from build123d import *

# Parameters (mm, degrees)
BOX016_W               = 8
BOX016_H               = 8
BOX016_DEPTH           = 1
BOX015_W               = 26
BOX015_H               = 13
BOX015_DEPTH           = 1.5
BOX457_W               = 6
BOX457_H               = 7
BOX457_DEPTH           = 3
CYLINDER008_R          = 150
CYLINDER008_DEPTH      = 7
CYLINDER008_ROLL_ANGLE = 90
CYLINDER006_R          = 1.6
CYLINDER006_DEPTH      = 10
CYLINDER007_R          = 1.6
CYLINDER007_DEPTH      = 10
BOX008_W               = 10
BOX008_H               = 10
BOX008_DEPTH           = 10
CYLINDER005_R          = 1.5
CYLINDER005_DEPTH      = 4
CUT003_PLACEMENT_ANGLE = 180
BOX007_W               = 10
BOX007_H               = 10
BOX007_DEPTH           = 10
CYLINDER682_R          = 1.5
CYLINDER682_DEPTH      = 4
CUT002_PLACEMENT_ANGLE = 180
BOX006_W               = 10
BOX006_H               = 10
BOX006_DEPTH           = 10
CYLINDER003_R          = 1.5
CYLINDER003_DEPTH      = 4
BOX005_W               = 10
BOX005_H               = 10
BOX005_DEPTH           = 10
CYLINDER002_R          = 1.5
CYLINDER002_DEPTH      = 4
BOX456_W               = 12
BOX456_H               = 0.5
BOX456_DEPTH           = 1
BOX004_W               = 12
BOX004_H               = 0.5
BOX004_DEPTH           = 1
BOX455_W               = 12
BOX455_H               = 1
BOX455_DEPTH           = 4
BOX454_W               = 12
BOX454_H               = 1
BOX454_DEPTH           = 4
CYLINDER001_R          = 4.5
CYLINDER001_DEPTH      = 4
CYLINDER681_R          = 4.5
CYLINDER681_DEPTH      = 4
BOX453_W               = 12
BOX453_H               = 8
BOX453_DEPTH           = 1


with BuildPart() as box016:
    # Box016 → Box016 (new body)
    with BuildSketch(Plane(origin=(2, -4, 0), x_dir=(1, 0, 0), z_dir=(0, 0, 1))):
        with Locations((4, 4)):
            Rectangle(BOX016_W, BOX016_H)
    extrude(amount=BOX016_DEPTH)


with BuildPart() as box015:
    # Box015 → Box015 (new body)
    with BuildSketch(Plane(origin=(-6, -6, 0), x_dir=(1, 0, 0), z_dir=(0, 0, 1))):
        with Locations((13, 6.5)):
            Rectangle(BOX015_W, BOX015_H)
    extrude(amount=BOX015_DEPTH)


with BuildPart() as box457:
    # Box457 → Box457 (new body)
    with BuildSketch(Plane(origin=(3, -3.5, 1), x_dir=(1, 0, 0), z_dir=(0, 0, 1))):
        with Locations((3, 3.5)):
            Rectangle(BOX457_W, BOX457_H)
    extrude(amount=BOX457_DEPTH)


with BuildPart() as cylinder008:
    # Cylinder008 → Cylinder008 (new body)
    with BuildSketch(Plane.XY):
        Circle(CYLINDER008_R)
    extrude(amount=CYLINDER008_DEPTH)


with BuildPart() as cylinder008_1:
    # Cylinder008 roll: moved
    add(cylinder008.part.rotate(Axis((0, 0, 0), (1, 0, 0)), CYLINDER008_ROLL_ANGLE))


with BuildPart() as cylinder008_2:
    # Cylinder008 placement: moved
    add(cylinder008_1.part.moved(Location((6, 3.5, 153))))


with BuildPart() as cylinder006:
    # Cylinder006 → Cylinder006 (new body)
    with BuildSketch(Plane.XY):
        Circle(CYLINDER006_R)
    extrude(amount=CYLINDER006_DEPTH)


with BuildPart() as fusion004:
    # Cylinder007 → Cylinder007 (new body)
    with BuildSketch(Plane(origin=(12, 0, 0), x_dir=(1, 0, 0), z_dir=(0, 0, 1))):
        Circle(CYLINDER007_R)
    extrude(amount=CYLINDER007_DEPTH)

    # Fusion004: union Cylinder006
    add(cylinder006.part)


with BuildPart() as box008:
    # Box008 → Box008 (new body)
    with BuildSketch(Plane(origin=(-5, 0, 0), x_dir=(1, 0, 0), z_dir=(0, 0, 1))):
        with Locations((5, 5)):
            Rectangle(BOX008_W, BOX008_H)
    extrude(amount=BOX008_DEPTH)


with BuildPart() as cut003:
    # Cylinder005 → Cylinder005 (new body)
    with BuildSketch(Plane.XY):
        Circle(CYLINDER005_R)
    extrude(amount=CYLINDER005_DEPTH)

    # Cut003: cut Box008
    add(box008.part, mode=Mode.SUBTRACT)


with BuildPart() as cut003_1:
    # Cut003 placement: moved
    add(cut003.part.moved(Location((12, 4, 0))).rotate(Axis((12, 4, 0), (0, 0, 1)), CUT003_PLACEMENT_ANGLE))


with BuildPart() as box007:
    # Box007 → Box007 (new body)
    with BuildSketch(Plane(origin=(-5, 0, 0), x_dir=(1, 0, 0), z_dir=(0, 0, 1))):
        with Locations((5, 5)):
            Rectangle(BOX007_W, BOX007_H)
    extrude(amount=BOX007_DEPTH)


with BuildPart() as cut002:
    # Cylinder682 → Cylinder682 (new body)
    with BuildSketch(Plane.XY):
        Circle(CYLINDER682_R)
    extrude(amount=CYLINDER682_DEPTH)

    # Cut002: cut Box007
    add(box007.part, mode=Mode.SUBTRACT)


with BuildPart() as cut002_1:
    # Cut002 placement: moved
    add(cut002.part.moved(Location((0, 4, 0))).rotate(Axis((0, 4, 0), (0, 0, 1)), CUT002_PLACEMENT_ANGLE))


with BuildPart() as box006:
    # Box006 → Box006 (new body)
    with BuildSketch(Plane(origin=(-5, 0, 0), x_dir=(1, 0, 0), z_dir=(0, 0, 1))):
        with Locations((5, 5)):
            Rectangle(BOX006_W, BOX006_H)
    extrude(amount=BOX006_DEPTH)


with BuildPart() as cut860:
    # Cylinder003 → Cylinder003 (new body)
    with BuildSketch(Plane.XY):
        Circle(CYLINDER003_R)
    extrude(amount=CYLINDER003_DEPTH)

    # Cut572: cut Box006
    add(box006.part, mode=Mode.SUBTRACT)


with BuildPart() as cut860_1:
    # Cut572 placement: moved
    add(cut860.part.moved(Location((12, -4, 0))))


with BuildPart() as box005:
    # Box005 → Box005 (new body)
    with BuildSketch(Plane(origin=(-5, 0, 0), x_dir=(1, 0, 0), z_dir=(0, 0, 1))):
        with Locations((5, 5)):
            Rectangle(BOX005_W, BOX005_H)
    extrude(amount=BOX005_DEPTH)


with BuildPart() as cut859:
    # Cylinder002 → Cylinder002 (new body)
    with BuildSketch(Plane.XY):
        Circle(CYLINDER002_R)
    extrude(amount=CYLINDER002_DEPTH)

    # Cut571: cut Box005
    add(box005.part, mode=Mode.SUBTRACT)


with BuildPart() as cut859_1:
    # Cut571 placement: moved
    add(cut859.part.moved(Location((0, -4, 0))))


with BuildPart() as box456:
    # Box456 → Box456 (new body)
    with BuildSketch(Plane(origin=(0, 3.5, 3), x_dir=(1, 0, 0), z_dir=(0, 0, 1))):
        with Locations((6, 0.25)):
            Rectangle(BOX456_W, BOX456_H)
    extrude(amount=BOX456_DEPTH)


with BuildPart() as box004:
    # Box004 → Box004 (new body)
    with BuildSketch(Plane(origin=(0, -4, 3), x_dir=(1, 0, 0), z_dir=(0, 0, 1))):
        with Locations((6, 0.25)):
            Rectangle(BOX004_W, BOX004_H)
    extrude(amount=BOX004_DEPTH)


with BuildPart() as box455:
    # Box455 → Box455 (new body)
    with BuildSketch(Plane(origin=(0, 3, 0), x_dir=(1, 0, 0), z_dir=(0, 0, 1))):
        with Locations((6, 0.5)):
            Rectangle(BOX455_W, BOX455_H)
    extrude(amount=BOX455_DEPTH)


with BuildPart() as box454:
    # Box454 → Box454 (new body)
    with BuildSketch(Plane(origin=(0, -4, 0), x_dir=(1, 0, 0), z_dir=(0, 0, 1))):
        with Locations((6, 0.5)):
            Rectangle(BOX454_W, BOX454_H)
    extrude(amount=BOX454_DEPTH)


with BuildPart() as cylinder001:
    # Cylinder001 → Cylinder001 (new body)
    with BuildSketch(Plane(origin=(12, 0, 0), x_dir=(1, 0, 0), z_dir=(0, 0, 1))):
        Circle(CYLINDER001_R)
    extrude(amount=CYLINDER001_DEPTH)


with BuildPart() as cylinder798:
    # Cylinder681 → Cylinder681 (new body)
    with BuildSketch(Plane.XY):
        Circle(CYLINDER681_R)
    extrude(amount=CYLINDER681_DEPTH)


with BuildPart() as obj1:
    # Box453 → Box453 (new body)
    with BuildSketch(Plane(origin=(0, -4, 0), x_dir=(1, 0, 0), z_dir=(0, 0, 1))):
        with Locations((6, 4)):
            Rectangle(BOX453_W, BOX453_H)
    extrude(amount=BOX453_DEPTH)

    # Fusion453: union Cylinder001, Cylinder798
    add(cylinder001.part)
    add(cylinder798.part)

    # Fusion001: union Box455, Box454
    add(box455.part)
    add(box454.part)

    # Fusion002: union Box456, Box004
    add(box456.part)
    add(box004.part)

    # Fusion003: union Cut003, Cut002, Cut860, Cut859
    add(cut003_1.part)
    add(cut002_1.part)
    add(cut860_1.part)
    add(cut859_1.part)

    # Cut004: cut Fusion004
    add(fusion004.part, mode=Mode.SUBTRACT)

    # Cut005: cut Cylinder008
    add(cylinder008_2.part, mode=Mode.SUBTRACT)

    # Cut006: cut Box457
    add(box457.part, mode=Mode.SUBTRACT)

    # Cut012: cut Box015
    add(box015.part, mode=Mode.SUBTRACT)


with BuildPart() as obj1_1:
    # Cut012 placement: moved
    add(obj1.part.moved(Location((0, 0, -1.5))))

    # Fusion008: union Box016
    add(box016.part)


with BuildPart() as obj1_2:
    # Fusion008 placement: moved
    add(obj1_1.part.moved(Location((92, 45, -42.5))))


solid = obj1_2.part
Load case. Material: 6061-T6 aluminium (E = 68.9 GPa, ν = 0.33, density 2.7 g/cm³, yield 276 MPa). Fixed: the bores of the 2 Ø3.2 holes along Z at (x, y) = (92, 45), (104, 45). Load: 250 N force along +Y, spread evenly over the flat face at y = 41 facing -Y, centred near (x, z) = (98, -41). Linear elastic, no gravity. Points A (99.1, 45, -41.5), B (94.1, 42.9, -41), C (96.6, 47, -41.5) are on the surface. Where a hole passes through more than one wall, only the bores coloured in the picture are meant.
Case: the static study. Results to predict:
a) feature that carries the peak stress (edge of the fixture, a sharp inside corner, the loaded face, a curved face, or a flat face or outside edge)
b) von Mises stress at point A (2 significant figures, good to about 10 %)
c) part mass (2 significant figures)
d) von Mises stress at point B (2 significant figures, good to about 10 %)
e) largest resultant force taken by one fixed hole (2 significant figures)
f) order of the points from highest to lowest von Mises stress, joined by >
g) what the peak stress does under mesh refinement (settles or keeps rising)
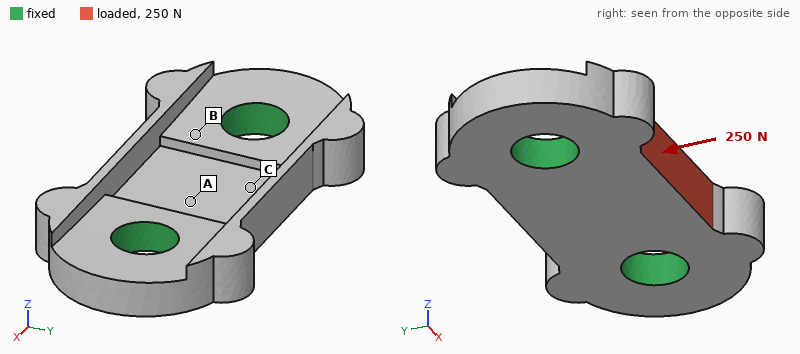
a sharp inside corner
28 MPa
0.69 g
60 MPa
130 N
B > A > C
keeps rising
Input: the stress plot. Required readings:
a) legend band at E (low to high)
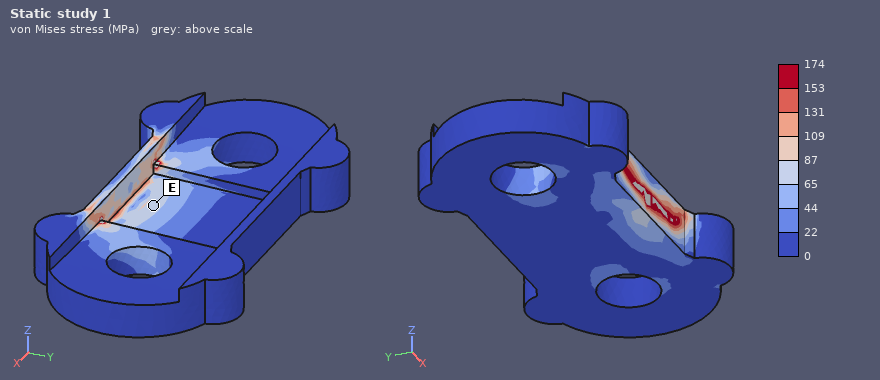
65 to 87 MPa
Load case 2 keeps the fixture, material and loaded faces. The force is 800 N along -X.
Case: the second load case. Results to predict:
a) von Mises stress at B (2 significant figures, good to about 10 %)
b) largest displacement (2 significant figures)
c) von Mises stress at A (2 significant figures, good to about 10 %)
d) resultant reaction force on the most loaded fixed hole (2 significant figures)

55 MPa
11 µm
31 MPa
440 N
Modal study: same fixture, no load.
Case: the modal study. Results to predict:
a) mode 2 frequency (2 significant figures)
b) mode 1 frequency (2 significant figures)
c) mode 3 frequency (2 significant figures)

64 kHz
62 kHz
75 kHz
